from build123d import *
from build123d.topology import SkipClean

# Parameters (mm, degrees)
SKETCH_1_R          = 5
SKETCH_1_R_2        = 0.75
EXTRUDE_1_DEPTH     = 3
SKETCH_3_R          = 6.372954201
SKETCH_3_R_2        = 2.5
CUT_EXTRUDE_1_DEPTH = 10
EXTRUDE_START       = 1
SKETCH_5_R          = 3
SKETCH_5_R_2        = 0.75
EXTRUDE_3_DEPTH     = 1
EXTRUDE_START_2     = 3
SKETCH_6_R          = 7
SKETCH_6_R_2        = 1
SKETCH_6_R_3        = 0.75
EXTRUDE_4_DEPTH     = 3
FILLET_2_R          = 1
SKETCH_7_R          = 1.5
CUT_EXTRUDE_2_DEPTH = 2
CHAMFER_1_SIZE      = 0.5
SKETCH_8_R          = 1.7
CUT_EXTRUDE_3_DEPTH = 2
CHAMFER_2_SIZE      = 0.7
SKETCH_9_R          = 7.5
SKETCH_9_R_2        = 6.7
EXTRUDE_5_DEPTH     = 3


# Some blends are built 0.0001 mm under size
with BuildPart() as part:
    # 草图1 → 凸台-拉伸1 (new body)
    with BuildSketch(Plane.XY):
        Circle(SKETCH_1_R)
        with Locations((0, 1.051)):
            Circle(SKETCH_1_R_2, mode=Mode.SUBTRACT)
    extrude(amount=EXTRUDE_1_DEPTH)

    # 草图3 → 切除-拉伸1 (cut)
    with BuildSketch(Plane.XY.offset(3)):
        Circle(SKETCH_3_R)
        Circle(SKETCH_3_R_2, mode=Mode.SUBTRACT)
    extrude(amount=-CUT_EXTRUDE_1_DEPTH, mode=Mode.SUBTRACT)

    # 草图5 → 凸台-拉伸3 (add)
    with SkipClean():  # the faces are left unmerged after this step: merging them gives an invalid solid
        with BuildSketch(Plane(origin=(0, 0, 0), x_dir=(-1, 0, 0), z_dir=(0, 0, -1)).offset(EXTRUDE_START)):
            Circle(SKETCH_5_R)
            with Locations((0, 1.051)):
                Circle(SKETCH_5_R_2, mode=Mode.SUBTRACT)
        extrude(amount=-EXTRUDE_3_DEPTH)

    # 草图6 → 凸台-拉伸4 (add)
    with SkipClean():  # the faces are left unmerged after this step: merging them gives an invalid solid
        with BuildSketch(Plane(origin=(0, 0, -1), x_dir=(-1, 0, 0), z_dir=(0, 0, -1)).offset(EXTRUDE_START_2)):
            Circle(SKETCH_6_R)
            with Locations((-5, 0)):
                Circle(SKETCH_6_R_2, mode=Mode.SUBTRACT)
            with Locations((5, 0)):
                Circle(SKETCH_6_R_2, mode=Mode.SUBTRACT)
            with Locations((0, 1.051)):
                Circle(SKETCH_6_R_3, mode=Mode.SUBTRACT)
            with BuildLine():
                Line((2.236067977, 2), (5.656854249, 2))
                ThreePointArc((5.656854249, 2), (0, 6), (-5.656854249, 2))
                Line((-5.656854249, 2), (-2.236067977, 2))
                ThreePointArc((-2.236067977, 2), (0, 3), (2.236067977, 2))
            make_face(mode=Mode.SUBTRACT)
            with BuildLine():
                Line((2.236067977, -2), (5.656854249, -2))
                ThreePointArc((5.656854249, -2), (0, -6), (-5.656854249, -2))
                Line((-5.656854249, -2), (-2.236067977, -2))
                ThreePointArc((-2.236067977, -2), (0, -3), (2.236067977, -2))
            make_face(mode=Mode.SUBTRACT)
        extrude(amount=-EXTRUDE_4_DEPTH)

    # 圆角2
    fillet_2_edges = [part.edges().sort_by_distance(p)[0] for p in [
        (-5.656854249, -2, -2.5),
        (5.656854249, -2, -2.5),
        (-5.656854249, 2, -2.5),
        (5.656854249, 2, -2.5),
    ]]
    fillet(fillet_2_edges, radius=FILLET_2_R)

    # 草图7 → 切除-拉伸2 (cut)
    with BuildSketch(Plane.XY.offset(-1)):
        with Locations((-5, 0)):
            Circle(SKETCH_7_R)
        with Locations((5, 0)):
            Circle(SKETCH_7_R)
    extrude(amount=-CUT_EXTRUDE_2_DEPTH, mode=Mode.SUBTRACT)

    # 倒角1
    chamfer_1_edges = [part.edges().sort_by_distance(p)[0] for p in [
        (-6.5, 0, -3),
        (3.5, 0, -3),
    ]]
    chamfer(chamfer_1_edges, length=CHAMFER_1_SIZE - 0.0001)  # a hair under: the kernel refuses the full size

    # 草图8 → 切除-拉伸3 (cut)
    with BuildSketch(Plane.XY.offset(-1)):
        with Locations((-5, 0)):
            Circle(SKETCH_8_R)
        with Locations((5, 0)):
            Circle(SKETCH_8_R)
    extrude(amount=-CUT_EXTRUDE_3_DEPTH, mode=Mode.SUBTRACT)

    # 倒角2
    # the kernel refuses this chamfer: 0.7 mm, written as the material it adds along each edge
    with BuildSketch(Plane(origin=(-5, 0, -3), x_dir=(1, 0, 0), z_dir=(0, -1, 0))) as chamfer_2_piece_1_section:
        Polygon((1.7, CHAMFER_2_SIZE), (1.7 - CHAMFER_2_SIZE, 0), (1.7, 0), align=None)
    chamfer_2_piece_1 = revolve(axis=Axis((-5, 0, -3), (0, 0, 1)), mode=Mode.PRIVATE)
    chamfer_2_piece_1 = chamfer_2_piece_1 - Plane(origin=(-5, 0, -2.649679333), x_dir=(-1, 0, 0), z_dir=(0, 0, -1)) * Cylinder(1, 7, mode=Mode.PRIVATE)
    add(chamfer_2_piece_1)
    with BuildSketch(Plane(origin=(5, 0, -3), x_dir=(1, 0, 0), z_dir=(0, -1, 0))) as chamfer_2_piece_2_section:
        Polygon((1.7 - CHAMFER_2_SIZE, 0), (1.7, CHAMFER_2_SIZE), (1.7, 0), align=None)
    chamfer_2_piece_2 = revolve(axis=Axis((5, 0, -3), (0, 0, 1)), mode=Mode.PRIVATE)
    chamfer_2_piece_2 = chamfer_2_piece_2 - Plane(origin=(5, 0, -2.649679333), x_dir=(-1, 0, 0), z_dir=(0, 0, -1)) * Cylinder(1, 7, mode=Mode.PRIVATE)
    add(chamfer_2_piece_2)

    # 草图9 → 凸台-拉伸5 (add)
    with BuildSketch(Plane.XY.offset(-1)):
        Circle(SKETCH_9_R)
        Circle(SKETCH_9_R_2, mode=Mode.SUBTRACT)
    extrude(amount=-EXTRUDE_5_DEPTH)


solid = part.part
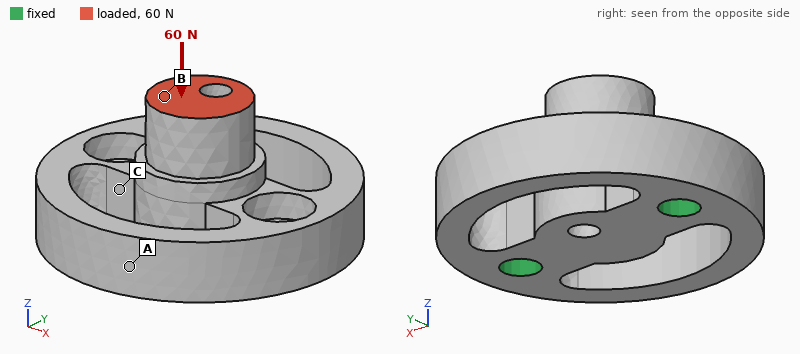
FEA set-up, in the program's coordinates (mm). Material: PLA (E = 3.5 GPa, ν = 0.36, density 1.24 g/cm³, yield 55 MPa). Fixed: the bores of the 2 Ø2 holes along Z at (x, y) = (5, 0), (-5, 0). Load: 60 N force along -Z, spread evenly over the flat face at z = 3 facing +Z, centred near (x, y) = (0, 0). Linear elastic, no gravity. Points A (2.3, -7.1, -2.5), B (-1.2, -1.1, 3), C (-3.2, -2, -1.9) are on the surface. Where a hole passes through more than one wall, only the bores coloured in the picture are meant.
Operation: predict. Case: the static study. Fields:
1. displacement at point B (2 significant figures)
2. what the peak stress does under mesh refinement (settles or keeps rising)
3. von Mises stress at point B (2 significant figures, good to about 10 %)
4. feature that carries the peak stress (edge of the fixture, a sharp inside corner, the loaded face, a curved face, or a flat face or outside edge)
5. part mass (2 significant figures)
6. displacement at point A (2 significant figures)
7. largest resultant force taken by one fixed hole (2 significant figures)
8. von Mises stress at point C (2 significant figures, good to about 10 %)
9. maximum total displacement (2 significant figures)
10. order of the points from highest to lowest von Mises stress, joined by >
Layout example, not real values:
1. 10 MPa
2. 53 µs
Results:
1. 16 µm
2. keeps rising
3. 3.5 MPa
4. edge of the fixture
5. 0.49 g
6. 7.1 µm
7. 36 N
8. 6.8 MPa
9. 17 µm
10. C > B > A
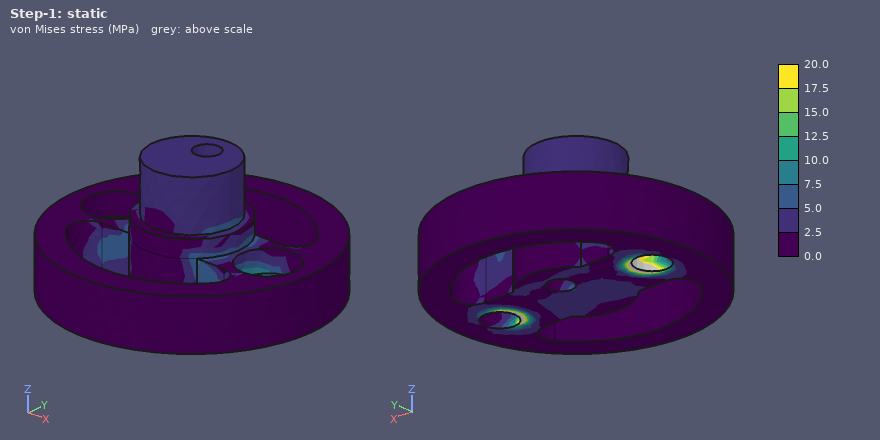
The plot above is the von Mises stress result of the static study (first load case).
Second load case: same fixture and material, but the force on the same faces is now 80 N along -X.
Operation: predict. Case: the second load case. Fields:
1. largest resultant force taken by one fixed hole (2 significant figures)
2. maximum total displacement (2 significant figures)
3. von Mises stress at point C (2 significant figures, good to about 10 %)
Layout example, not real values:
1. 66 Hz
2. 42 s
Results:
1. 71 N
2. 69 µm
3. 14 MPa
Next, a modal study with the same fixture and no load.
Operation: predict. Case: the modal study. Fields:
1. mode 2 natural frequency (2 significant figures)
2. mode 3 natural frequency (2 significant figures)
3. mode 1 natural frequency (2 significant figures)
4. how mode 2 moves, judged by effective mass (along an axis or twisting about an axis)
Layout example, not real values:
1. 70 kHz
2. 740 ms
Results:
1. 9100 Hz
2. 11 kHz
3. 6700 Hz
4. along Z
